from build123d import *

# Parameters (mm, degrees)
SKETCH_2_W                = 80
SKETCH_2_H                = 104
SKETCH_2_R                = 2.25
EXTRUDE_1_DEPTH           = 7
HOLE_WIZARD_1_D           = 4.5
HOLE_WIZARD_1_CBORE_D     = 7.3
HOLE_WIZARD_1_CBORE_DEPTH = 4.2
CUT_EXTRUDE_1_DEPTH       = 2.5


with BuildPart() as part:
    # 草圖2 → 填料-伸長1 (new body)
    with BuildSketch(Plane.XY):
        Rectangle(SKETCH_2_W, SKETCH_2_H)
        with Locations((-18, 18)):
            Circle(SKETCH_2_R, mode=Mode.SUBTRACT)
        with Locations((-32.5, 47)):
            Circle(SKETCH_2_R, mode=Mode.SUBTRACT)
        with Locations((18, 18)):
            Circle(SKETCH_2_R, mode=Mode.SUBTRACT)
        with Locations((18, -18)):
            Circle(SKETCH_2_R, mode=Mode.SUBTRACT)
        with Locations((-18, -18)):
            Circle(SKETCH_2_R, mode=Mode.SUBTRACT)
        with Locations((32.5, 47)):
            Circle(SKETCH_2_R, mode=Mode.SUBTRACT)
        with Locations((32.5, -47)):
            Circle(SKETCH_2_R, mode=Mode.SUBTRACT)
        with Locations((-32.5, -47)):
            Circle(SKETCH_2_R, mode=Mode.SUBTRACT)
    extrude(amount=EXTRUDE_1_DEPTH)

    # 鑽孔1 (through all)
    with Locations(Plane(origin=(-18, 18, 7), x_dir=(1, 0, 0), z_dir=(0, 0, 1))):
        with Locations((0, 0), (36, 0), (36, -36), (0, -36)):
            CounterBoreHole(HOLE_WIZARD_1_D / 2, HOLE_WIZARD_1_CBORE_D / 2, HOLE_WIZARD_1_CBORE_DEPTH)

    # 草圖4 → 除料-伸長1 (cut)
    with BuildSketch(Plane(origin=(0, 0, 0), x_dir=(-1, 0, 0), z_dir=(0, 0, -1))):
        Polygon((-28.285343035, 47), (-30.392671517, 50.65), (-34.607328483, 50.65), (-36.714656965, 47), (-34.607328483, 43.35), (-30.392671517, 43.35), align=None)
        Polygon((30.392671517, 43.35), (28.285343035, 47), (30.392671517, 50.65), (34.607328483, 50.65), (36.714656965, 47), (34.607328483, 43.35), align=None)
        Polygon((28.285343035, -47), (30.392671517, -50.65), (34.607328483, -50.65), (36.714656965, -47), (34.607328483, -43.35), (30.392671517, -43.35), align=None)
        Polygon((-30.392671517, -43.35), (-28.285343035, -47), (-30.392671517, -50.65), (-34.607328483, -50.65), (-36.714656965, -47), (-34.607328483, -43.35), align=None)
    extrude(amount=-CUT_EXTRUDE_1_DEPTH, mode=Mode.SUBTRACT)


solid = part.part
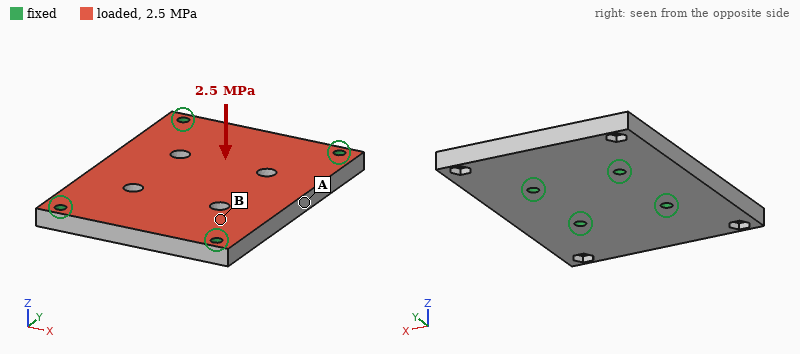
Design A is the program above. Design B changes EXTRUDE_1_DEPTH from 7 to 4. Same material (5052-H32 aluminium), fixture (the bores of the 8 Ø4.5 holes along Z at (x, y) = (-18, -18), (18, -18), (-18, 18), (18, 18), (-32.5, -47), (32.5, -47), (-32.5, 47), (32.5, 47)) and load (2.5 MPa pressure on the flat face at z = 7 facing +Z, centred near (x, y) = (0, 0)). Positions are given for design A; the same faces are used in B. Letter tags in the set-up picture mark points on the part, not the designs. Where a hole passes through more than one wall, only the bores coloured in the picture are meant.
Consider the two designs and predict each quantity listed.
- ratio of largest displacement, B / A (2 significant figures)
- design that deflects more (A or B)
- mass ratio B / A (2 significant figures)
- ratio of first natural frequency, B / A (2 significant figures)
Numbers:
5.0
B
0.57
0.65
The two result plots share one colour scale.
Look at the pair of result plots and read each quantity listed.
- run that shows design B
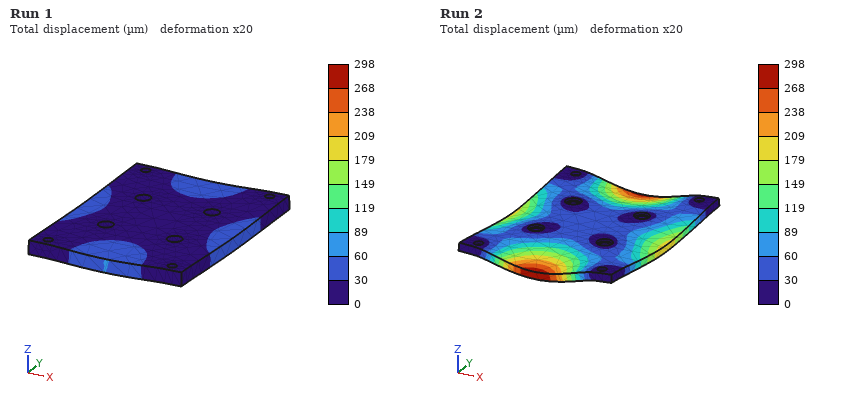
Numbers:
Run 2
